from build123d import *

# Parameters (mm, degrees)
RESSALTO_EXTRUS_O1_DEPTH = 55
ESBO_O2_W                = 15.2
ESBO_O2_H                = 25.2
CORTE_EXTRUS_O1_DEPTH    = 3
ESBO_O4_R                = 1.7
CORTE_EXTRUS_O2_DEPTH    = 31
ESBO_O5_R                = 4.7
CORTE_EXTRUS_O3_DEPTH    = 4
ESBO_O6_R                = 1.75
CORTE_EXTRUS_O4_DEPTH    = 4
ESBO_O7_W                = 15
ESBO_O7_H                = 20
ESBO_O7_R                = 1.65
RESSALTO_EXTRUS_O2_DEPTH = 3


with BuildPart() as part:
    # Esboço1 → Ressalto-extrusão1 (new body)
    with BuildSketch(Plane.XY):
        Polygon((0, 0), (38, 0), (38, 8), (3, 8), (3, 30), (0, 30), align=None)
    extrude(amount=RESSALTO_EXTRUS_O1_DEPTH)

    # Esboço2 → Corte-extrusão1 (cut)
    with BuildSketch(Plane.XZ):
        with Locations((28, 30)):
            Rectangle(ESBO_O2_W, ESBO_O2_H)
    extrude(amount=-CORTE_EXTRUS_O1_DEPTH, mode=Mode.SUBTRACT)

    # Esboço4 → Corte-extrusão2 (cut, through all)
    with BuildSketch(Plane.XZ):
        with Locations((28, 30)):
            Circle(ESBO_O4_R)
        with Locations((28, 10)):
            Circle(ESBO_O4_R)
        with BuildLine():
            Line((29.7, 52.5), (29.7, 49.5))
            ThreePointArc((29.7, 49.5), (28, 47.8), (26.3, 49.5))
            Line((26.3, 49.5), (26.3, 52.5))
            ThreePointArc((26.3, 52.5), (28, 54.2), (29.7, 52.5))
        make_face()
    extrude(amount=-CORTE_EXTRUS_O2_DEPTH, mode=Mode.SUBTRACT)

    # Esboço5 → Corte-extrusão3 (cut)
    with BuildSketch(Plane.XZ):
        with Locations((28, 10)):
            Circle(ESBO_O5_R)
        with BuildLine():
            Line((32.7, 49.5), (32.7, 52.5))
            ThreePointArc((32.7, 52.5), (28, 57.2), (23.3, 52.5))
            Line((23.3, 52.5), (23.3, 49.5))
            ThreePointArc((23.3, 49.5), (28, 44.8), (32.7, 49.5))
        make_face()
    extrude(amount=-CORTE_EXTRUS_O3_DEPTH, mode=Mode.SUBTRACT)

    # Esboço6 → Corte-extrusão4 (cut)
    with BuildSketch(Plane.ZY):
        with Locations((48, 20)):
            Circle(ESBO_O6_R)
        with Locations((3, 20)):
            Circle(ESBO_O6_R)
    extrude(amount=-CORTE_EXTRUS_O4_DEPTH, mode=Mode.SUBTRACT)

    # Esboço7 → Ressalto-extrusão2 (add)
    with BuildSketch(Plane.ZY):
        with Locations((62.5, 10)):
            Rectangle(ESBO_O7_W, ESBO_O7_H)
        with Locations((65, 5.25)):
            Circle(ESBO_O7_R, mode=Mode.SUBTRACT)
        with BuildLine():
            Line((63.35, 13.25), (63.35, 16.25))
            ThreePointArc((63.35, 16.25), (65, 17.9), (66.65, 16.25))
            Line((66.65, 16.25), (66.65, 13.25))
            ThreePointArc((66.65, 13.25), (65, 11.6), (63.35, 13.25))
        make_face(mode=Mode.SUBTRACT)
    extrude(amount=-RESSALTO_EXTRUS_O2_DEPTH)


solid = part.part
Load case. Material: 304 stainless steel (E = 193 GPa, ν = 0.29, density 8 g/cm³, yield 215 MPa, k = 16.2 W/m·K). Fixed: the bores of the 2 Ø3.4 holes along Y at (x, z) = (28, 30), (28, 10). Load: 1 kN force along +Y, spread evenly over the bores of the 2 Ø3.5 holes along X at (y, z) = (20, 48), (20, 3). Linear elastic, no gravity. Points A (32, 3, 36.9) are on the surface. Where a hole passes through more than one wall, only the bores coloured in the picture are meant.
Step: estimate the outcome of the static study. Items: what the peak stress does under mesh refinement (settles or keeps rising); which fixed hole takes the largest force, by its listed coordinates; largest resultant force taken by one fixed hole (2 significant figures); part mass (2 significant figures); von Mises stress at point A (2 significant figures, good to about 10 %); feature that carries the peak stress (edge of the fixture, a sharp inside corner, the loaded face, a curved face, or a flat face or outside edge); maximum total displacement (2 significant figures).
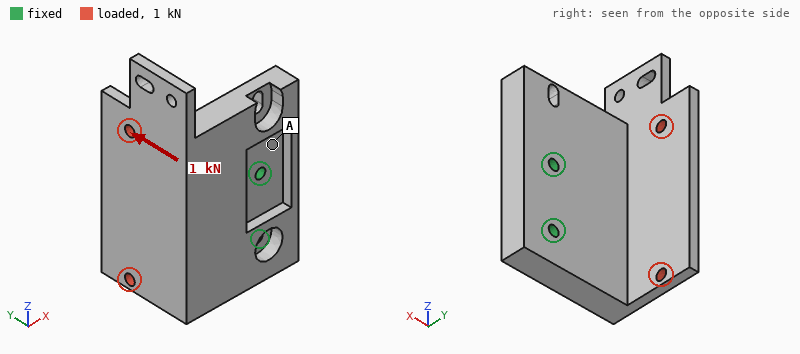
keeps rising
(28, 30)
710 N
150 g
39 MPa
edge of the fixture
95 µm
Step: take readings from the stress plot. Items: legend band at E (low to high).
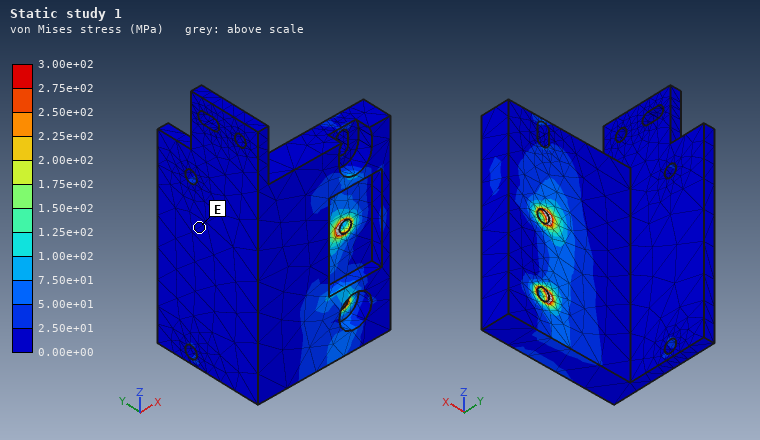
0.00e+00 to 2.50e+01 MPa
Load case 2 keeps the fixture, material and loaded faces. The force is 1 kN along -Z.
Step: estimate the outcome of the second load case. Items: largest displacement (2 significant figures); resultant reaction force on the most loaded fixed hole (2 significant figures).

51 µm
1.4 kN
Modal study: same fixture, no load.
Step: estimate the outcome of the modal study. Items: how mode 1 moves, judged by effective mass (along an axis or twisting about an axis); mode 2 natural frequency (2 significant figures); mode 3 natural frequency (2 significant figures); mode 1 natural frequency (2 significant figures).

along Y
3500 Hz
4900 Hz
2100 Hz
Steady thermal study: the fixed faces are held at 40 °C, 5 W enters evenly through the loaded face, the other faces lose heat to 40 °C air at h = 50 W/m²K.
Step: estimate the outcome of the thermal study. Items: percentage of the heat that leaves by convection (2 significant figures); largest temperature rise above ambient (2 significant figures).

77 %
46 K
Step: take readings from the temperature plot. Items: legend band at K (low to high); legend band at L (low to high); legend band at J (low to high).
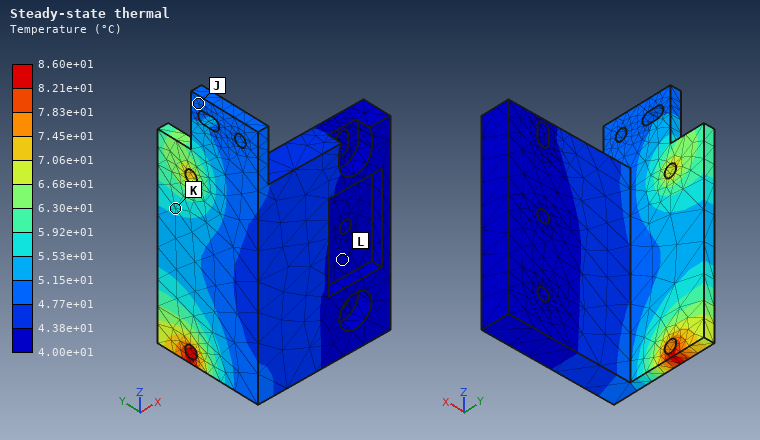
5.53e+01 to 5.92e+01 °C
4.00e+01 to 4.38e+01 °C
4.77e+01 to 5.15e+01 °C
